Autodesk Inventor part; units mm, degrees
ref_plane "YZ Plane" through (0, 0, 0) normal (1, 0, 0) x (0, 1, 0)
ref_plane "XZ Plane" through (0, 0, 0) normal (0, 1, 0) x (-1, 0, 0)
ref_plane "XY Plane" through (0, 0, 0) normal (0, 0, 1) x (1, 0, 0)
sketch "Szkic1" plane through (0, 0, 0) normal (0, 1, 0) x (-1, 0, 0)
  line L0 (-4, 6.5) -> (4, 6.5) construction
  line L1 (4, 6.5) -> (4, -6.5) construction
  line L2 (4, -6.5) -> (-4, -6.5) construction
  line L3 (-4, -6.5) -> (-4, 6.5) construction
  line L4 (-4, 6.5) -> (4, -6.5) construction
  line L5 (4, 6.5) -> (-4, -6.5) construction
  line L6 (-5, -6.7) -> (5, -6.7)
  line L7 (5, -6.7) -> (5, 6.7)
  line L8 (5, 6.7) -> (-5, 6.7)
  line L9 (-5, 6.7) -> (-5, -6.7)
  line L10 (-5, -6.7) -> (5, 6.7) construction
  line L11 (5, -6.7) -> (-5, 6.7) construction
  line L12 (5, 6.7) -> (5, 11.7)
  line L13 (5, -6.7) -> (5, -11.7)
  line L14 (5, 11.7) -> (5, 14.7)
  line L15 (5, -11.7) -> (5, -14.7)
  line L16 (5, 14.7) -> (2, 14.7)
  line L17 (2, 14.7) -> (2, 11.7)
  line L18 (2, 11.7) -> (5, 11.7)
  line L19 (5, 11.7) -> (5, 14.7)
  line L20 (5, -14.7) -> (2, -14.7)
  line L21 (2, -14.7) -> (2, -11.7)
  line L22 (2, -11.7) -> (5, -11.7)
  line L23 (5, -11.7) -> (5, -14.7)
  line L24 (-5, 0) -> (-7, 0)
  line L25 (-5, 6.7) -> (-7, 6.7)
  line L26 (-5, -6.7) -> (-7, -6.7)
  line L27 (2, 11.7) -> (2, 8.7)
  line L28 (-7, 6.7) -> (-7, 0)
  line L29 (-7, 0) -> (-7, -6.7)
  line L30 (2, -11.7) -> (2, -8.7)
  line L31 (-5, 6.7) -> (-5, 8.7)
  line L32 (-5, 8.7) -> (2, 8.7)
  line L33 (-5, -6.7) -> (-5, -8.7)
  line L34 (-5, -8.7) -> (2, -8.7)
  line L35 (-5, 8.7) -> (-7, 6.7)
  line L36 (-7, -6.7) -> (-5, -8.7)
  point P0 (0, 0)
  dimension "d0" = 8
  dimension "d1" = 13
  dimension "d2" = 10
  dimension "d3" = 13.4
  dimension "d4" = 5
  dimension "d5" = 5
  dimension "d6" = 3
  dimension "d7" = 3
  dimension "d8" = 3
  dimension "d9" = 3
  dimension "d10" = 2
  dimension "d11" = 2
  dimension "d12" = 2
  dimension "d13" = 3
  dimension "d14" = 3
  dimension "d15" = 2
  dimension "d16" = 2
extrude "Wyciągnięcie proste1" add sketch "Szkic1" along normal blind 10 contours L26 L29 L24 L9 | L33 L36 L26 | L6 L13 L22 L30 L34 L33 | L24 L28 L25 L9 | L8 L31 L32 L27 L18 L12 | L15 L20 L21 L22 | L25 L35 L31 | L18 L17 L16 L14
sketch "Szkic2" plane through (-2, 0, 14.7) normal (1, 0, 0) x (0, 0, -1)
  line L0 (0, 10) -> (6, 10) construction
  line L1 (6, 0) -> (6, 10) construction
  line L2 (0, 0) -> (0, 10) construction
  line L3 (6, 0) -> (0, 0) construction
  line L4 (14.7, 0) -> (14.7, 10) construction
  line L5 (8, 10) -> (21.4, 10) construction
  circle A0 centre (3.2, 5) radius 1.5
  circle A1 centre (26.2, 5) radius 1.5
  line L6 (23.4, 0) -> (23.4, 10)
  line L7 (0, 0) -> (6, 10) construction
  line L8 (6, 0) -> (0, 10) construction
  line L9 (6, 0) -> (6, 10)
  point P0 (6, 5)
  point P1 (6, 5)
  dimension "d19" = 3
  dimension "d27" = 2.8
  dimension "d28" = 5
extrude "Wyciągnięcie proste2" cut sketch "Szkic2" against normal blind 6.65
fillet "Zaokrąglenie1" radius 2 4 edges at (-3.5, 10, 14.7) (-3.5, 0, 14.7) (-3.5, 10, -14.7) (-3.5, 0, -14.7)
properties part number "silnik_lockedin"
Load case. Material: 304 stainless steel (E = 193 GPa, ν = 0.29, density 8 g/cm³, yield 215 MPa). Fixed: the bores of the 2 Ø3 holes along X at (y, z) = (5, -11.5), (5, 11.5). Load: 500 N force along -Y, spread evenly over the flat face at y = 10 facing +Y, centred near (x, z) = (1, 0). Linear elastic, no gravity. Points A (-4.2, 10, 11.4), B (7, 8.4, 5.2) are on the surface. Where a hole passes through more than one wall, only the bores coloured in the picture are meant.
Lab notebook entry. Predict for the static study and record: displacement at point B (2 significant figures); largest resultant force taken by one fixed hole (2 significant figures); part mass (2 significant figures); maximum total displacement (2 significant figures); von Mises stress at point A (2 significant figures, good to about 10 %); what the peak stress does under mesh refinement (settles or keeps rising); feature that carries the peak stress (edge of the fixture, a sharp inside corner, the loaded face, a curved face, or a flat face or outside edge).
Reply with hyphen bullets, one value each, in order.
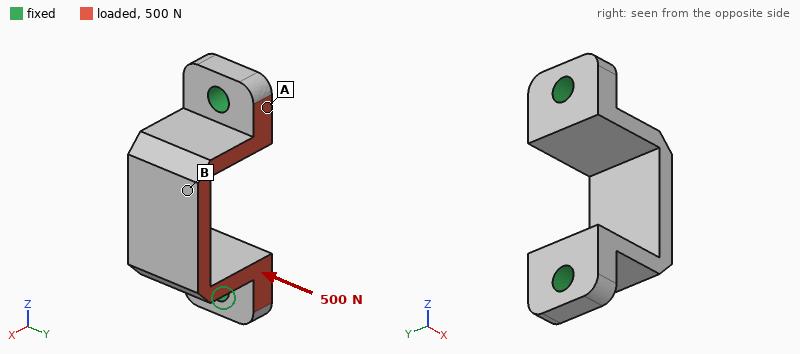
- 8.2 µm
- 250 N
- 8.1 g
- 8.7 µm
- 21 MPa
- keeps rising
- edge of the fixture
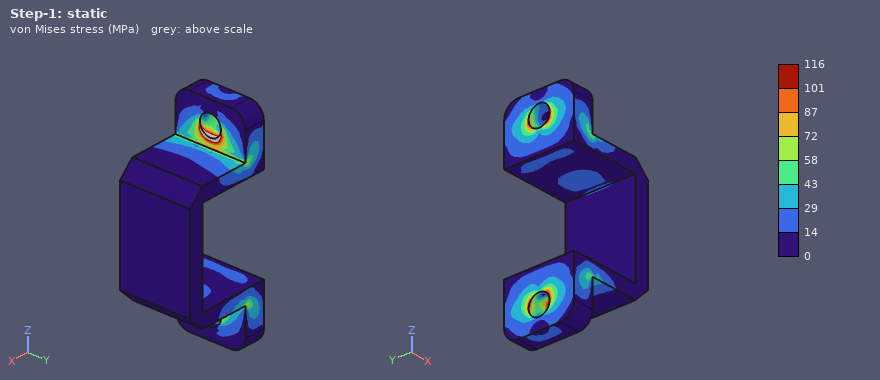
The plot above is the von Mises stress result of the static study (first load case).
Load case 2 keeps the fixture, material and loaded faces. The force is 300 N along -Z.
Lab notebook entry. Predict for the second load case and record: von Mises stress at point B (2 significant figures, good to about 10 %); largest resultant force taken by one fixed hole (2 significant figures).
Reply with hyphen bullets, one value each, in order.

- 22 MPa
- 160 N
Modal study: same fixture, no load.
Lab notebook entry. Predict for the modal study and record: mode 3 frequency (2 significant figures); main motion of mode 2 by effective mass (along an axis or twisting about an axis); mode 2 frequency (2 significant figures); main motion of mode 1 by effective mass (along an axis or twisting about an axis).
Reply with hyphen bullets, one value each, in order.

- 23 kHz
- along Y
- 16 kHz
- along Z
